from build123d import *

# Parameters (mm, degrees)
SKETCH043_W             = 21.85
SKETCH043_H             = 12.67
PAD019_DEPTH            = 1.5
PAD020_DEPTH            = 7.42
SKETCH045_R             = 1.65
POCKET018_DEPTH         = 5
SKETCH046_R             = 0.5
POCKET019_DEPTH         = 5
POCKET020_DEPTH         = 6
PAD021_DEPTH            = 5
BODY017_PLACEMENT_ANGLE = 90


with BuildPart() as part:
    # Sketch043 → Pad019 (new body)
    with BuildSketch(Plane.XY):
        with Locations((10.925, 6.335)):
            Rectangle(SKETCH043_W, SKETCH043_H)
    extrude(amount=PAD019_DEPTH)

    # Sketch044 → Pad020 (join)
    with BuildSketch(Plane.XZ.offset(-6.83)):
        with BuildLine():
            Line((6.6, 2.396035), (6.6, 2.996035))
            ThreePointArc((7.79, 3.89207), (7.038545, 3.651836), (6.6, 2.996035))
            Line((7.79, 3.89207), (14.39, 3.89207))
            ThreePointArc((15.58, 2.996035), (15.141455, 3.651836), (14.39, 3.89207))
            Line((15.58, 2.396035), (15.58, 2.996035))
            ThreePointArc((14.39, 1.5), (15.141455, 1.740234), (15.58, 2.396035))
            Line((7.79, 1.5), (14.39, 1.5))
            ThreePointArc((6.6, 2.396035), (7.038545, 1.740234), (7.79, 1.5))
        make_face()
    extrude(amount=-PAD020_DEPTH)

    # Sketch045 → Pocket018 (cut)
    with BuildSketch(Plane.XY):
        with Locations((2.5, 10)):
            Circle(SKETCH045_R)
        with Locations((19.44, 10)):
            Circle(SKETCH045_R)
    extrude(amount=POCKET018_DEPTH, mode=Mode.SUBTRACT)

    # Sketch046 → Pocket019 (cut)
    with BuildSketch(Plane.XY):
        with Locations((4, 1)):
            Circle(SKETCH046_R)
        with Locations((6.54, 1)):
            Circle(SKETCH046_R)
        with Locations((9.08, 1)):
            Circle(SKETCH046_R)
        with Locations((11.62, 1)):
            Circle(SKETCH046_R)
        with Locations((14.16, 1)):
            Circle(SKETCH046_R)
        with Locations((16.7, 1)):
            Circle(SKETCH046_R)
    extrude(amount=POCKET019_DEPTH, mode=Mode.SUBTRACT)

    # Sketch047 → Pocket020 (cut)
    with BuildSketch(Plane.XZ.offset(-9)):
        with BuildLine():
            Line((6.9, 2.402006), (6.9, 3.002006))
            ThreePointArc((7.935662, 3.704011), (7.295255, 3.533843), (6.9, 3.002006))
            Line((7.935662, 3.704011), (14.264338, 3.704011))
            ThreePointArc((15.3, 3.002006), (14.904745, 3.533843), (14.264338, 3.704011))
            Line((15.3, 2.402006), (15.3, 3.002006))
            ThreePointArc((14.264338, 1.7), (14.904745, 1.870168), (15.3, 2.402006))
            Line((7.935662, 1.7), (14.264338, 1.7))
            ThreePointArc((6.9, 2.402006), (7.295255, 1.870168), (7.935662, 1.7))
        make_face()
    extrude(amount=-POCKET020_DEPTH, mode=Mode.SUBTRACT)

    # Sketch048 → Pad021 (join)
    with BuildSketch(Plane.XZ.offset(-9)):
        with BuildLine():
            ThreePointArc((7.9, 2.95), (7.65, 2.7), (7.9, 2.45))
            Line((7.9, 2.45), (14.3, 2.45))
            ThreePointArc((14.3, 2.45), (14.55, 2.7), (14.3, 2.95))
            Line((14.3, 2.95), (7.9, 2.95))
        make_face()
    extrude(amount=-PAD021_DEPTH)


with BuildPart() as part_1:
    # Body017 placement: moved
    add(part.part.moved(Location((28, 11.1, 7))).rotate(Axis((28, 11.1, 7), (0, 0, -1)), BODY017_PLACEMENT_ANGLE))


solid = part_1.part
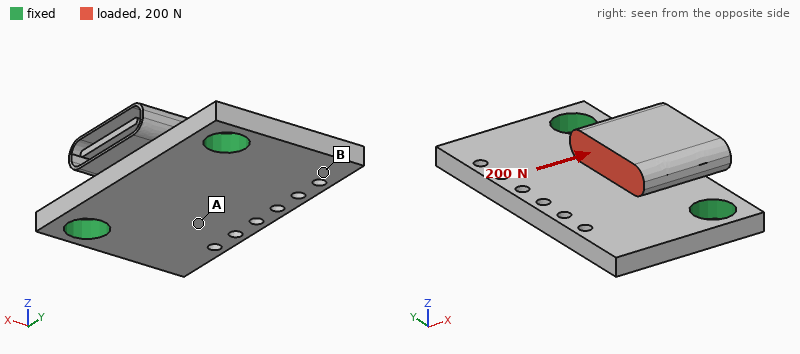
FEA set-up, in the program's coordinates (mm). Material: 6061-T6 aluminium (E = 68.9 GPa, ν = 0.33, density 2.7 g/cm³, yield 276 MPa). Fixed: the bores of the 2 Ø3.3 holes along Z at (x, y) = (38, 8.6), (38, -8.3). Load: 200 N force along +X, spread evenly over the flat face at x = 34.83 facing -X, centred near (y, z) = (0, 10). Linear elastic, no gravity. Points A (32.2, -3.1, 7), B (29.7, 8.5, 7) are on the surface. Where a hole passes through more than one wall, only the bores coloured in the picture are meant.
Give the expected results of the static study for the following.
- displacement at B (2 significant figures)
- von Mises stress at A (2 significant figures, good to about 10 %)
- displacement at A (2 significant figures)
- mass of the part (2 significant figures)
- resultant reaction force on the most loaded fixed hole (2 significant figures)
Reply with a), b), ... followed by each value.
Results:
a) 11 µm
b) 18 MPa
c) 12 µm
d) 1.3 g
e) 110 N
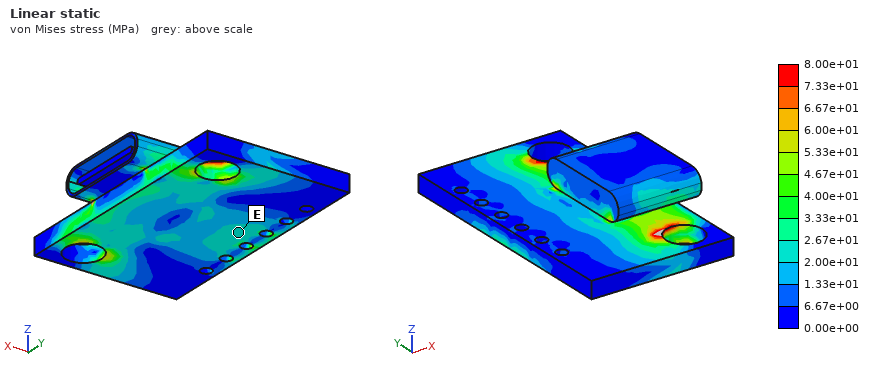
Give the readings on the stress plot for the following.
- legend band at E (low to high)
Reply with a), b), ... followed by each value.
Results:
a) 2.00e+01 to 2.67e+01 MPa
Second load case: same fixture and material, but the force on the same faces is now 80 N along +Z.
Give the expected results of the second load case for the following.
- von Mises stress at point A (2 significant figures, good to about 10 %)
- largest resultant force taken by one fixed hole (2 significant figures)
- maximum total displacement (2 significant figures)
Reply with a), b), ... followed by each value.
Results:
a) 12 MPa
b) 42 N
c) 15 µm
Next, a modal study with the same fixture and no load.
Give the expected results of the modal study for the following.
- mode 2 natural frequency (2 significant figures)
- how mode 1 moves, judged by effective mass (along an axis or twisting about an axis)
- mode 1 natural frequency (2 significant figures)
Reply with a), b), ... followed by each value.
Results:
a) 15 kHz
b) along Z
c) 13 kHz
